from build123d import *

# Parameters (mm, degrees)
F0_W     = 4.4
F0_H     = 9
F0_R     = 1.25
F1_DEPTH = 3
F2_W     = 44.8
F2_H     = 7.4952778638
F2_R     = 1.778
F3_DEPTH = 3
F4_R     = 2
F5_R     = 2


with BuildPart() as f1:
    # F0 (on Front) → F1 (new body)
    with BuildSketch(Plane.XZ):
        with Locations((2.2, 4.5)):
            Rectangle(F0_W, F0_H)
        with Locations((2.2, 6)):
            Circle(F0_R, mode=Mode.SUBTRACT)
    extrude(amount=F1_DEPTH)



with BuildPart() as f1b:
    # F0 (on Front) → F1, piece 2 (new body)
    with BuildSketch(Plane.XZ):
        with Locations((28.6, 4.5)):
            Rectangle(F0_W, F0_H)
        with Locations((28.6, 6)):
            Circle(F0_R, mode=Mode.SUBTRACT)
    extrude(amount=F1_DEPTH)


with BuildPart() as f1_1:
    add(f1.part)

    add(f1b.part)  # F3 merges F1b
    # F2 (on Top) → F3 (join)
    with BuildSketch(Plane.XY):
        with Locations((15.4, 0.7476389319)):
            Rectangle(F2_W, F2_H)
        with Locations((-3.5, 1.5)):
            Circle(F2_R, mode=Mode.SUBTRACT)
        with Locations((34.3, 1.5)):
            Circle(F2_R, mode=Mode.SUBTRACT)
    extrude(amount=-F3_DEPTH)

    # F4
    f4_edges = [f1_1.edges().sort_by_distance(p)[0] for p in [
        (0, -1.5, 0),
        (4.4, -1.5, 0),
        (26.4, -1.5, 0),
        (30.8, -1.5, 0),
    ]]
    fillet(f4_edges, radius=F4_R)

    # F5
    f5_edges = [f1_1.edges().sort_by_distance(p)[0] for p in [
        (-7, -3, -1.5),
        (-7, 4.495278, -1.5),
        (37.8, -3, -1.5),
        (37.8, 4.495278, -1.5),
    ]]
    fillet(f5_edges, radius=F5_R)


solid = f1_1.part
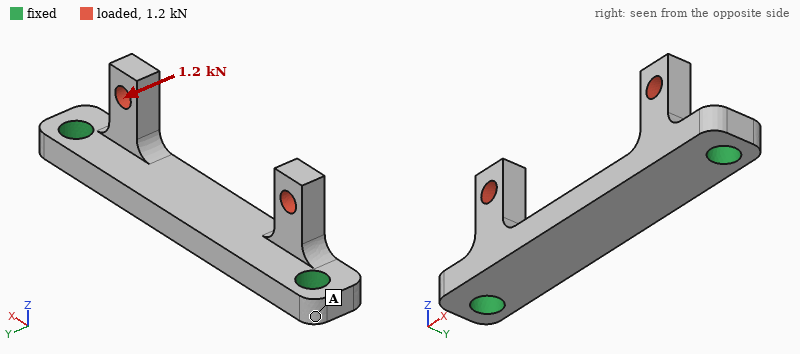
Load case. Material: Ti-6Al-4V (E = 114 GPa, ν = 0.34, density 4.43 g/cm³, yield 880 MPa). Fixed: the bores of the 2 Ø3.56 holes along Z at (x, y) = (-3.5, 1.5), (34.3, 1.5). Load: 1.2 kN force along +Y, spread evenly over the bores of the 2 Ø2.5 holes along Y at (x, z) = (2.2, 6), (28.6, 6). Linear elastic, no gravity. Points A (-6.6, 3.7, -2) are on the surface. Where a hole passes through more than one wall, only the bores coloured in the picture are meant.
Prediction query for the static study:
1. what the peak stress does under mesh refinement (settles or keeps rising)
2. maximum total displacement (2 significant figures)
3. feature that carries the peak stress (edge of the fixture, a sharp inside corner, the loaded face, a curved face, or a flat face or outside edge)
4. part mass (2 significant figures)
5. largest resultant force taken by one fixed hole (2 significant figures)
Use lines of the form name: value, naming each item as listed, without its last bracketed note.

what the peak stress does under mesh refinement: keeps rising
maximum total displacement: 0.19 mm
feature that carries the peak stress: a sharp inside corner
part mass: 5.1 g
largest resultant force taken by one fixed hole: 600 N
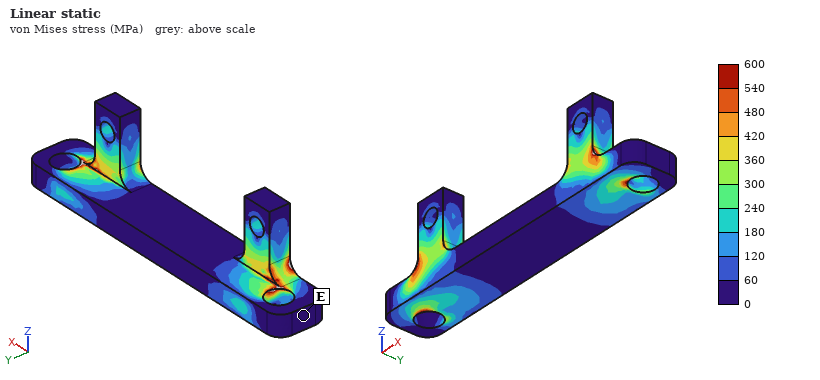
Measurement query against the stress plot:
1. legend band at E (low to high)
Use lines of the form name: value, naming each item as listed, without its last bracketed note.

legend band at E: 0 to 60 MPa
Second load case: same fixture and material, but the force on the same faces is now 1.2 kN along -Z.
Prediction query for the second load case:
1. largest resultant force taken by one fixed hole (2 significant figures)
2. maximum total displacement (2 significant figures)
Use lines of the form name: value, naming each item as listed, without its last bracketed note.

largest resultant force taken by one fixed hole: 600 N
maximum total displacement: 50 µm
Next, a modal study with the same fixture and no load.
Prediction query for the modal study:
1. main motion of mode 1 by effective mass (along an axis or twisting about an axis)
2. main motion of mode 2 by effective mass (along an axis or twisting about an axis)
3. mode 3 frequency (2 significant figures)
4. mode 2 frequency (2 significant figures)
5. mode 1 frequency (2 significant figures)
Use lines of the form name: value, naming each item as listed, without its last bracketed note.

main motion of mode 1 by effective mass: along Z
main motion of mode 2 by effective mass: along Y
mode 3 frequency: 20 kHz
mode 2 frequency: 18 kHz
mode 1 frequency: 11 kHz
